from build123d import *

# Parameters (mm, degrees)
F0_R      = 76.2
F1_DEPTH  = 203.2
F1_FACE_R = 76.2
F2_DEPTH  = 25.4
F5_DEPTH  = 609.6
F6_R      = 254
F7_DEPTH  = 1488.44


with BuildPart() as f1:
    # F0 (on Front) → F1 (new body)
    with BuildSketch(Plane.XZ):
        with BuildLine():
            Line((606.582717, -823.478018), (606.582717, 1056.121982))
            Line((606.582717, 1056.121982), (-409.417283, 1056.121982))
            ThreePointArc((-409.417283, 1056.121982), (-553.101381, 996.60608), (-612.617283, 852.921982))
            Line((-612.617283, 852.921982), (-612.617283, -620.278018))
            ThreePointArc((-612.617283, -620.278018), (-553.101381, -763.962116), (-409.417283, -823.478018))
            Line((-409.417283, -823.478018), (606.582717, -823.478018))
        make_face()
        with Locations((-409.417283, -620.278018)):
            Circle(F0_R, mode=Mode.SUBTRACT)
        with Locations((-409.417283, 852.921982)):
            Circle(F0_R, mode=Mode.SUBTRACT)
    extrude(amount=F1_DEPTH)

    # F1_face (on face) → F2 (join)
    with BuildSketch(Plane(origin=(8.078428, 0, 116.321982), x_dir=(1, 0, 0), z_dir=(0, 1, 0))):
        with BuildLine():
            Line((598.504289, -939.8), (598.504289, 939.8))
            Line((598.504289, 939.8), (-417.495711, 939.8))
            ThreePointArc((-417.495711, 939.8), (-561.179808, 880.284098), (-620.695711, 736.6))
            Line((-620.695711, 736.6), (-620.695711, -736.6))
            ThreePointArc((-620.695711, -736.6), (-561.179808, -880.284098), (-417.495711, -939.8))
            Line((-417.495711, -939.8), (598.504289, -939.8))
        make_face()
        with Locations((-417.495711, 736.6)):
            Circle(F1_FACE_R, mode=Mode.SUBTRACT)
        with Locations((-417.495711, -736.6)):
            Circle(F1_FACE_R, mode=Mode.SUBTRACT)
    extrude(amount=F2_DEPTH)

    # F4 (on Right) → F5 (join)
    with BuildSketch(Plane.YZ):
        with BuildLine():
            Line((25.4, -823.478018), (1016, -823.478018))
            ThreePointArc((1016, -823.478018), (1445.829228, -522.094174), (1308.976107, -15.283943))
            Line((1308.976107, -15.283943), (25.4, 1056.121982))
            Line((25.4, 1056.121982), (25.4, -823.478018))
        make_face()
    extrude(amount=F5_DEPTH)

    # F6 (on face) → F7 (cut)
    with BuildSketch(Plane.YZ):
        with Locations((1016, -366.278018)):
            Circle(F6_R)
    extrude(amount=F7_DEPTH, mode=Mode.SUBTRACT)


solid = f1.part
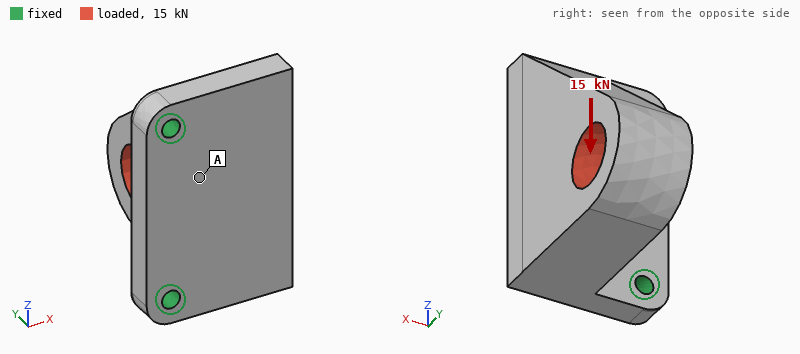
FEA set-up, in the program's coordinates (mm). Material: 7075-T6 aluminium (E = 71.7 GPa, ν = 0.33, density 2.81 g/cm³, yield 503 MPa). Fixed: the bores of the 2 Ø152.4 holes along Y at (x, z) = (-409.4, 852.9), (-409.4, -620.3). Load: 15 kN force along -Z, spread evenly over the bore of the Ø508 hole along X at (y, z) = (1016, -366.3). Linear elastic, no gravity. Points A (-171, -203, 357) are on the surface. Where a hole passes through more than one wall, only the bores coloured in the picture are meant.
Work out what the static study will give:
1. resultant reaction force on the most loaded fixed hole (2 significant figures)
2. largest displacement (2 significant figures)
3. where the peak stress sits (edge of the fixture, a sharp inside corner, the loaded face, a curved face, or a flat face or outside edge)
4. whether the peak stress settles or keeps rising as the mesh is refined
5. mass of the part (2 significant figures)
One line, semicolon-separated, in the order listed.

15 kN; 16 µm; edge of the fixture; keeps rising; 4200 kg
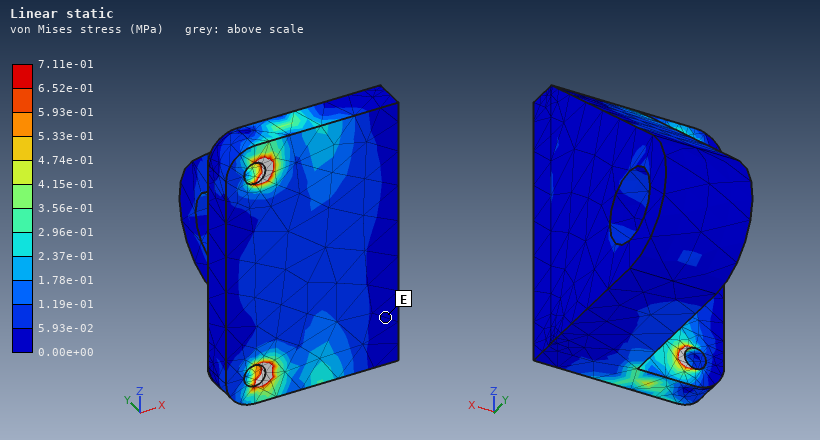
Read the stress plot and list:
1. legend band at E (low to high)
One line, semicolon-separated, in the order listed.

0.00e+00 to 5.93e-02 MPa
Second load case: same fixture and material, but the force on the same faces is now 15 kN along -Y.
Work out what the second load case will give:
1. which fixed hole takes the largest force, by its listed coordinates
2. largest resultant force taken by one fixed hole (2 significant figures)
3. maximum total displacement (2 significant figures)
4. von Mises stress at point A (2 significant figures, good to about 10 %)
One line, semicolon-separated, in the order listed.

(-409.4, -620.3); 12 kN; 65 µm; 0.25 MPa
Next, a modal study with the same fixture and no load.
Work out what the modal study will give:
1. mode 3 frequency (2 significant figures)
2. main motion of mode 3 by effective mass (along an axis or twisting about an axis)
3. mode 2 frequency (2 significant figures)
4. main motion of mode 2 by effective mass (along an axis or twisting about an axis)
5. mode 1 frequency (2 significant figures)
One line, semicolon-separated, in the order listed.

210 Hz; along Y; 140 Hz; along Z; 45 Hz
